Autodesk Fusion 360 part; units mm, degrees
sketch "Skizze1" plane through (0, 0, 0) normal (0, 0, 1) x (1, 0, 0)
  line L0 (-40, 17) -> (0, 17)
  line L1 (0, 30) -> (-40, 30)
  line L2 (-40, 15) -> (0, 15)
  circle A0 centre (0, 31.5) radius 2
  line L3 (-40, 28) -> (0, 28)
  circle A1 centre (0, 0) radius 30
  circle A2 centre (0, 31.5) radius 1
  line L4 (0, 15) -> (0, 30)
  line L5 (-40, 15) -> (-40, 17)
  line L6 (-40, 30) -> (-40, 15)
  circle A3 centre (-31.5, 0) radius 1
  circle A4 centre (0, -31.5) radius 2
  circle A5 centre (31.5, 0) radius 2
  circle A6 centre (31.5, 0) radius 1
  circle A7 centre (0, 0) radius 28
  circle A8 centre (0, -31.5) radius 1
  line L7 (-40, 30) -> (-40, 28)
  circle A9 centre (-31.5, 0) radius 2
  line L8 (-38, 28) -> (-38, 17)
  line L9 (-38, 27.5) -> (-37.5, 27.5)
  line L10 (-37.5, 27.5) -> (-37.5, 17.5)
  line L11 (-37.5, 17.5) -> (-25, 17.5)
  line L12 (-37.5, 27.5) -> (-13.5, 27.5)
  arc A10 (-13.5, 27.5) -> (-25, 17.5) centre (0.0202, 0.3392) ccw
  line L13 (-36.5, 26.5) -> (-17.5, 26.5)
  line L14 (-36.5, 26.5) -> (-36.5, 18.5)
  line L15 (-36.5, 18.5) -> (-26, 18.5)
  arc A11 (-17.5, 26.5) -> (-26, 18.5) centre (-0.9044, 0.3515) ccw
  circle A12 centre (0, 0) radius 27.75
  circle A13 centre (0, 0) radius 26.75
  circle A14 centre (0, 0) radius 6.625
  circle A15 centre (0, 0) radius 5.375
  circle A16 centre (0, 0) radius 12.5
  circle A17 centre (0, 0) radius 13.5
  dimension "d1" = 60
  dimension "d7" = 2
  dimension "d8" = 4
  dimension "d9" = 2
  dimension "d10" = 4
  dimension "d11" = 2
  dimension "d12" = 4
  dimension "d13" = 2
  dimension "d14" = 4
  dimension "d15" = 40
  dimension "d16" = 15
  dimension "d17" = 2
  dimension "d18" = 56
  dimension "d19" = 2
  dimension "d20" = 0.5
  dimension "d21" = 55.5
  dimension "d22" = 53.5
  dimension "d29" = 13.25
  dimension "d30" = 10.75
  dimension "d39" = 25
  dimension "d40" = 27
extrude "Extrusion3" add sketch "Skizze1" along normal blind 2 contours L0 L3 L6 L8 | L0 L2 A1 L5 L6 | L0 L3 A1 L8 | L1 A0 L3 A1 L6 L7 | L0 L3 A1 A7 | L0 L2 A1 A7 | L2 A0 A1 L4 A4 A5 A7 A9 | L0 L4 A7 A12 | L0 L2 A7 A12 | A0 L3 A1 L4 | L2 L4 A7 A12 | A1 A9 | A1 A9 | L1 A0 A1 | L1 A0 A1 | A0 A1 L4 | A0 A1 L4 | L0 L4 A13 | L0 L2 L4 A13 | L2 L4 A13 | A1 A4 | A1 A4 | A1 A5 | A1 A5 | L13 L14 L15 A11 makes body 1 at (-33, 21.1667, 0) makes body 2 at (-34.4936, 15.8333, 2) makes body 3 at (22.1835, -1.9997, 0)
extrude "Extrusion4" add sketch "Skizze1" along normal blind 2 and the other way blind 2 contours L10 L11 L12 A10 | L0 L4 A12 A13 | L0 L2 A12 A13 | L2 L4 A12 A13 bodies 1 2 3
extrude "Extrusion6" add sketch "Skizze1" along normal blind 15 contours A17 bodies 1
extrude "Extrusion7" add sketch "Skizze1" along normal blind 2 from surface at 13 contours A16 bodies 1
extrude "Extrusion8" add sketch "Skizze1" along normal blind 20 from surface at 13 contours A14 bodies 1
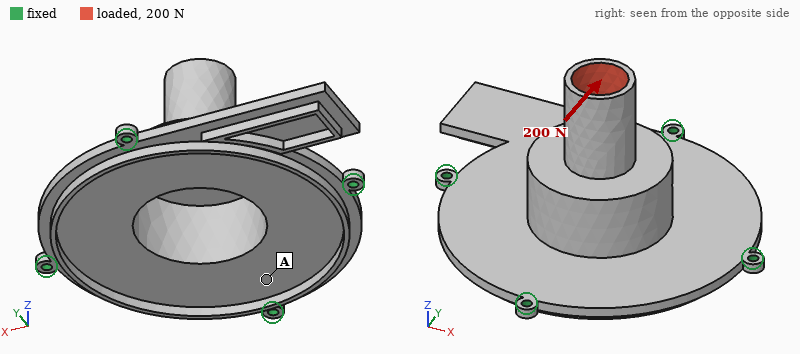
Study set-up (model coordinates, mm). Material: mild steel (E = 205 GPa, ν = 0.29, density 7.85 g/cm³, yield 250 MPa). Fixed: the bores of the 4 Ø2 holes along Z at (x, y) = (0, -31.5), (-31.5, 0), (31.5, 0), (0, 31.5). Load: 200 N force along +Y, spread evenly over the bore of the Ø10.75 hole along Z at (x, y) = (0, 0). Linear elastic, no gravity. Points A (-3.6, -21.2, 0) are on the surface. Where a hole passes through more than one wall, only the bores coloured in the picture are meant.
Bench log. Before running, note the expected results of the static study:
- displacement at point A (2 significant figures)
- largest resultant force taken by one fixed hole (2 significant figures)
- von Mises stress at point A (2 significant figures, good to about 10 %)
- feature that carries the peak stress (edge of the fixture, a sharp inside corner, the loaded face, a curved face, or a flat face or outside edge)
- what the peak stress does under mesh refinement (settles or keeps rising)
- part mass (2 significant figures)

10 µm
100 N
13 MPa
edge of the fixture
keeps rising
67 g
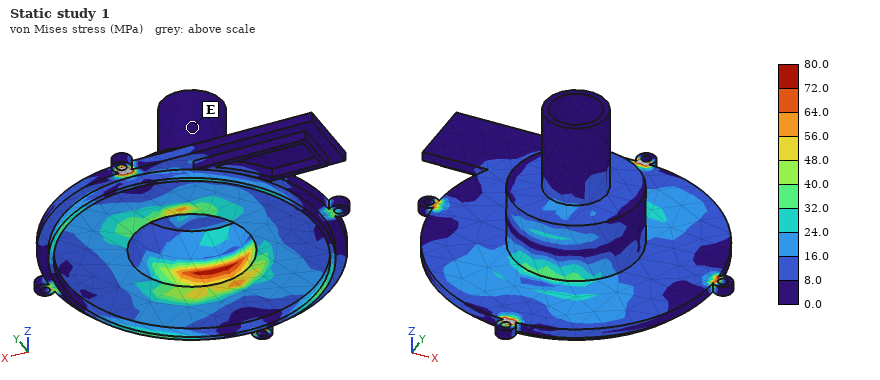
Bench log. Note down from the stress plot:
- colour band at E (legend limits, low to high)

0.0 to 8.0 MPa
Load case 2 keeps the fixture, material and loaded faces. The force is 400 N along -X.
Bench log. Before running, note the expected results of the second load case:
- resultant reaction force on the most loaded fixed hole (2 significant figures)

200 N
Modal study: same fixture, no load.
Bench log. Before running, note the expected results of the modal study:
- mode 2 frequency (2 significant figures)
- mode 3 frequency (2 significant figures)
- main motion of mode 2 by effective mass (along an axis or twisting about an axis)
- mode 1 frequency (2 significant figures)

2900 Hz
3200 Hz
along Z
2000 Hz
